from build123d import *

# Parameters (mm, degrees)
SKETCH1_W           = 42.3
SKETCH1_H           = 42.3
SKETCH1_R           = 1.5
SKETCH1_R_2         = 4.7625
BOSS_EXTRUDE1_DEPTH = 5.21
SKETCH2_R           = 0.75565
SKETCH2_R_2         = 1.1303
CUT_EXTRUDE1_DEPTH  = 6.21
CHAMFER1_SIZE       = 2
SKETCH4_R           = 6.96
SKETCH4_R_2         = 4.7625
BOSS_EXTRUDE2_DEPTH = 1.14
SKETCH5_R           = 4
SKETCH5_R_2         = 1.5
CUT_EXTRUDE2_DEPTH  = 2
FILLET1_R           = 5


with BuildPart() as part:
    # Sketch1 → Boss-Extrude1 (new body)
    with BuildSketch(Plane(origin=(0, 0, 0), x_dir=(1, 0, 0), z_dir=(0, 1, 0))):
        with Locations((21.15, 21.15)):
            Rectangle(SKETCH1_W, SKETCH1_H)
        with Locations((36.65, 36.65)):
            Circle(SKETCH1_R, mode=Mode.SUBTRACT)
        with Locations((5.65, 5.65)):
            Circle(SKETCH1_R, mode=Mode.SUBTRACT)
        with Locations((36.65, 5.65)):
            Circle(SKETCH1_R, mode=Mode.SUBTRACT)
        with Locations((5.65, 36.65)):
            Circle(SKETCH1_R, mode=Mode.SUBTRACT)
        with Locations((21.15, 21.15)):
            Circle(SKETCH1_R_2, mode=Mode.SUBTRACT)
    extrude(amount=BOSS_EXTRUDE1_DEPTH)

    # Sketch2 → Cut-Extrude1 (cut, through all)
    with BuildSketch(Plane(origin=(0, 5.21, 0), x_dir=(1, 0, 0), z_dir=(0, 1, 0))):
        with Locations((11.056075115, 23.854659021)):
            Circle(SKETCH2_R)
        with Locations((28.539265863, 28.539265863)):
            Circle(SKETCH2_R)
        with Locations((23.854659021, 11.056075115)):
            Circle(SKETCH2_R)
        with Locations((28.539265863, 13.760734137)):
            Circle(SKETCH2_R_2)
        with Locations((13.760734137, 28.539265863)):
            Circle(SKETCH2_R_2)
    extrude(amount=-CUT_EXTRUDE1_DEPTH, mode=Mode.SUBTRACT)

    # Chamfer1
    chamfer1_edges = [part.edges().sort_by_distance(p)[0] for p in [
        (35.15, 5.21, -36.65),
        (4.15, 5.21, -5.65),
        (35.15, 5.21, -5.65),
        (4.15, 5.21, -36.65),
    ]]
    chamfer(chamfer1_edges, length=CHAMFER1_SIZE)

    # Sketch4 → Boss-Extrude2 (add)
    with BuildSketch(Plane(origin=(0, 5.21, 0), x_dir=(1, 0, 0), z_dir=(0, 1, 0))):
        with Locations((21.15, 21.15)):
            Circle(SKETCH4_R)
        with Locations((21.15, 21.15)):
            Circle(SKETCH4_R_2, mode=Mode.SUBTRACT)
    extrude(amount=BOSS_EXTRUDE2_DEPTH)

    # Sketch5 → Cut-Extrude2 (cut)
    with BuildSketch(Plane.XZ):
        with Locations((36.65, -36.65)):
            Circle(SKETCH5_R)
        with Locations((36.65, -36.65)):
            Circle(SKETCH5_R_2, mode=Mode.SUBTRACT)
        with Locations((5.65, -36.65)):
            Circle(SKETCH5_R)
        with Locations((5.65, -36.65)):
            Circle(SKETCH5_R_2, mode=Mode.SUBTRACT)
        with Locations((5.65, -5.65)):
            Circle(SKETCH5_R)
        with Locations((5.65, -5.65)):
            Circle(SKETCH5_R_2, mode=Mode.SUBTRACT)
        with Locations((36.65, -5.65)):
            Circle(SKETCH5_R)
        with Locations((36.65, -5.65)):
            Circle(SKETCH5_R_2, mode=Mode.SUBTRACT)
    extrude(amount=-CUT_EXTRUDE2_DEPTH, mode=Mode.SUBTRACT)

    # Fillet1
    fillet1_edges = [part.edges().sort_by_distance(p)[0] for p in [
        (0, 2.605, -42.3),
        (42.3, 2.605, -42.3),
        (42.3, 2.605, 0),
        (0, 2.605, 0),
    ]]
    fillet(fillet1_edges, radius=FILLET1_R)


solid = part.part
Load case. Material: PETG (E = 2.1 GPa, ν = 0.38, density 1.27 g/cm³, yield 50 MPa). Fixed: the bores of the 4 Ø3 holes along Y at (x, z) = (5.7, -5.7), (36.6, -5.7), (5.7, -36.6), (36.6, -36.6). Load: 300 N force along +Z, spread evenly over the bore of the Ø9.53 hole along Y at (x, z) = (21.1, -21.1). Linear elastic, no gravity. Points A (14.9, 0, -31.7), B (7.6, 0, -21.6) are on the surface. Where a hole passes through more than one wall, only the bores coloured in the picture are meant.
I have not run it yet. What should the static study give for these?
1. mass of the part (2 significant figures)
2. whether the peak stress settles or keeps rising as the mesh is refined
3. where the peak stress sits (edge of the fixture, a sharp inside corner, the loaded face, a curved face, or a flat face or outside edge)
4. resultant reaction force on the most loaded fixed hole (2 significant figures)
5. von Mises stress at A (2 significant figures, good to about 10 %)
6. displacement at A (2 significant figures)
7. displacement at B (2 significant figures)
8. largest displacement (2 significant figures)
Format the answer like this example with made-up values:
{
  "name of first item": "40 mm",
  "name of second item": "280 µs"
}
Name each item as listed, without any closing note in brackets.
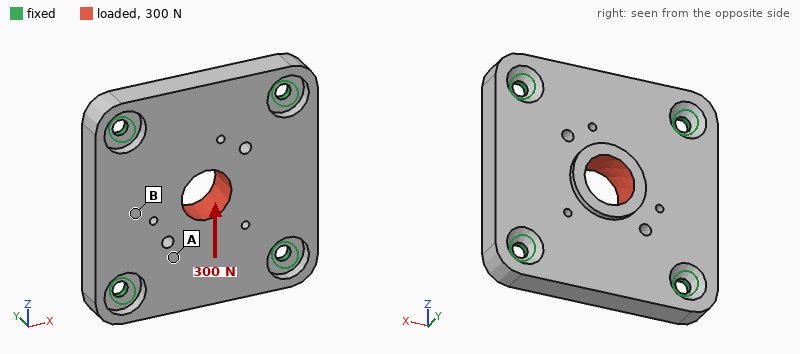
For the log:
{
  "mass of the part": "10 g",
  "whether the peak stress settles or keeps rising as the mesh is refined": "keeps rising",
  "where the peak stress sits": "edge of the fixture",
  "resultant reaction force on the most loaded fixed hole": "80 N",
  "von Mises stress at A": "1.5 MPa",
  "displacement at A": "17 µm",
  "displacement at B": "11 µm",
  "largest displacement": "28 µm"
}
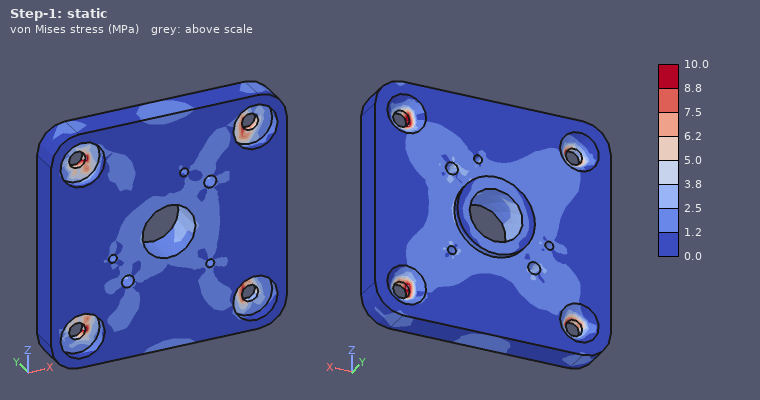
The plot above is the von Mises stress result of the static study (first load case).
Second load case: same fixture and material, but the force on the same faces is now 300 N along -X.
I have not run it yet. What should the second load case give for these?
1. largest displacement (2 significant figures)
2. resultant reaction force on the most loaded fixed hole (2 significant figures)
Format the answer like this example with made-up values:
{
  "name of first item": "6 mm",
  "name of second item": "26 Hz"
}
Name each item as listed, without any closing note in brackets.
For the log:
{
  "largest displacement": "28 µm",
  "resultant reaction force on the most loaded fixed hole": "80 N"
}
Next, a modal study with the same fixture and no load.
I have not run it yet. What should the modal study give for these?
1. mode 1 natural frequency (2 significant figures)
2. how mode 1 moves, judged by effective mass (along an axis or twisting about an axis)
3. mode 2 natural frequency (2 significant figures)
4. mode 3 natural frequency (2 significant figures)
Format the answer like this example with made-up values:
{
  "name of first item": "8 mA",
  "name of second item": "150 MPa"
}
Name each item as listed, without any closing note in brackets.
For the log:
{
  "mode 1 natural frequency": "3000 Hz",
  "how mode 1 moves, judged by effective mass": "along Y",
  "mode 2 natural frequency": "4000 Hz",
  "mode 3 natural frequency": "4300 Hz"
}
